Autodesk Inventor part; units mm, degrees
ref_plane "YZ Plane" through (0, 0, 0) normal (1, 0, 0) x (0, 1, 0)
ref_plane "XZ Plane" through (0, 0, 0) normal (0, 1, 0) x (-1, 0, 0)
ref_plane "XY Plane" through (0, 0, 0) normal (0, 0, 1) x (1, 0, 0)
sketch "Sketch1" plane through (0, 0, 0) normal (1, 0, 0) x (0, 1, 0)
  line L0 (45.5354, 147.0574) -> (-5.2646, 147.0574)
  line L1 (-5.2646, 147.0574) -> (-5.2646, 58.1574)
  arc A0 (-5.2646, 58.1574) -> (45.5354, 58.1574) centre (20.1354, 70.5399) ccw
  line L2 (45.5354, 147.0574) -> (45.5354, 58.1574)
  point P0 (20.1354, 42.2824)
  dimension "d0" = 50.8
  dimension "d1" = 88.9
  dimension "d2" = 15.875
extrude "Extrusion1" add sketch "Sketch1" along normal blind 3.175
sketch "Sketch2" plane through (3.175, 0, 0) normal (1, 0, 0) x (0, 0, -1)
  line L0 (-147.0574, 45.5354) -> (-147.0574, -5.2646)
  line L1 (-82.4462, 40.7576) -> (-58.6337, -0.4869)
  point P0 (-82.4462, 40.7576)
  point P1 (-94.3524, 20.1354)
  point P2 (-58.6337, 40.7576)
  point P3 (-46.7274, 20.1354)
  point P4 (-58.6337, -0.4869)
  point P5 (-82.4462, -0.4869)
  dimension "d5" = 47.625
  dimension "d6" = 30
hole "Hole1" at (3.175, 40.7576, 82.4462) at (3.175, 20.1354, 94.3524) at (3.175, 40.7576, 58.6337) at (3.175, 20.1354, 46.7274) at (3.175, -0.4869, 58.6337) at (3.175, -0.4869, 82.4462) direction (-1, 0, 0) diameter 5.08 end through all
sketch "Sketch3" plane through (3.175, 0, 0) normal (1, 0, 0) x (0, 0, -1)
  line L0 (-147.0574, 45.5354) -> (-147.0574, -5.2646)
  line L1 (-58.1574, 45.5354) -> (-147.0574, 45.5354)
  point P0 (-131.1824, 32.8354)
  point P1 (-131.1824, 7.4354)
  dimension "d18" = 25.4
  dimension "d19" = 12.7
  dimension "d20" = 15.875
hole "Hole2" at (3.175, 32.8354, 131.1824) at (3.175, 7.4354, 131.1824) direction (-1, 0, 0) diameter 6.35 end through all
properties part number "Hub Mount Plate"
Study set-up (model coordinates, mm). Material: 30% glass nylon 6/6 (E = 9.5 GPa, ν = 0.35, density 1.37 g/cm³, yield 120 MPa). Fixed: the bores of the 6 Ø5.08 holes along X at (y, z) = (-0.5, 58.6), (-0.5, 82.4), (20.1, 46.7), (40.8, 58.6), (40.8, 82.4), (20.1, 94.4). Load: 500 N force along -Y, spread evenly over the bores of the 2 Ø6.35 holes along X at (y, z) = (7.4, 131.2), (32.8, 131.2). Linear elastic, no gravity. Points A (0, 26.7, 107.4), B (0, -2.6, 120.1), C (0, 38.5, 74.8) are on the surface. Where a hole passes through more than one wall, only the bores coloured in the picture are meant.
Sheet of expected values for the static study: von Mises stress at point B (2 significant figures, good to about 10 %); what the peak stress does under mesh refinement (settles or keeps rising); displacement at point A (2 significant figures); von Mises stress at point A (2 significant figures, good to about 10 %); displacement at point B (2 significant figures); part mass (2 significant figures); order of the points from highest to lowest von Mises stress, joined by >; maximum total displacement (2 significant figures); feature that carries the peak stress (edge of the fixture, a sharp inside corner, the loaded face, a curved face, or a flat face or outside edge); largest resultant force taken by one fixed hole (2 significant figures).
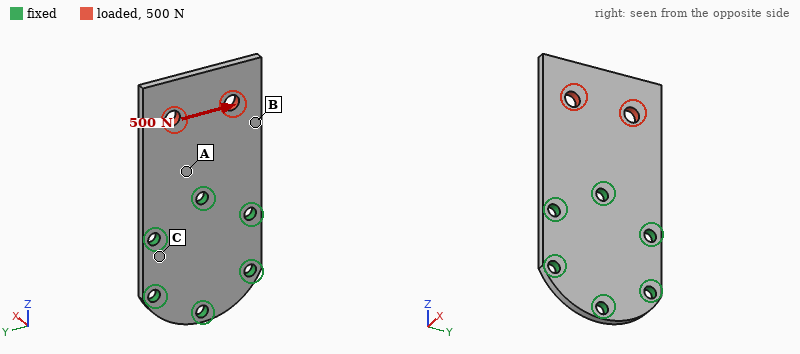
4.2 MPa
keeps rising
0.029 mm
7.5 MPa
0.072 mm
21 g
A > B > C
0.13 mm
edge of the fixture
440 N
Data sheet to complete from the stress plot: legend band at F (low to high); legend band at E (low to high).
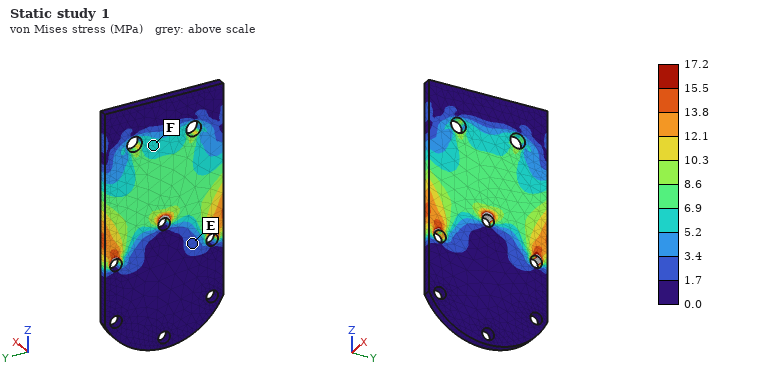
5.2 to 6.9 MPa
1.7 to 3.4 MPa
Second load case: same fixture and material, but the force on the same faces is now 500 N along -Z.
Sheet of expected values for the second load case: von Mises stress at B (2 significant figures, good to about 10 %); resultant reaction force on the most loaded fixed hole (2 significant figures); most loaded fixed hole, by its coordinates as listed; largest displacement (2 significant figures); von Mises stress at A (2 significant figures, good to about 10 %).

2.3 MPa
230 N
(20.1, 94.4)
18 µm
3.5 MPa
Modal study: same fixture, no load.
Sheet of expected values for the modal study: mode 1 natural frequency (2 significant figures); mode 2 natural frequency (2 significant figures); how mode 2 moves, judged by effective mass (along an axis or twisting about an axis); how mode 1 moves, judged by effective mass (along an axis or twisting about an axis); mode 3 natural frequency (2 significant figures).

480 Hz
1000 Hz
twisting about Z
along X
2500 Hz
